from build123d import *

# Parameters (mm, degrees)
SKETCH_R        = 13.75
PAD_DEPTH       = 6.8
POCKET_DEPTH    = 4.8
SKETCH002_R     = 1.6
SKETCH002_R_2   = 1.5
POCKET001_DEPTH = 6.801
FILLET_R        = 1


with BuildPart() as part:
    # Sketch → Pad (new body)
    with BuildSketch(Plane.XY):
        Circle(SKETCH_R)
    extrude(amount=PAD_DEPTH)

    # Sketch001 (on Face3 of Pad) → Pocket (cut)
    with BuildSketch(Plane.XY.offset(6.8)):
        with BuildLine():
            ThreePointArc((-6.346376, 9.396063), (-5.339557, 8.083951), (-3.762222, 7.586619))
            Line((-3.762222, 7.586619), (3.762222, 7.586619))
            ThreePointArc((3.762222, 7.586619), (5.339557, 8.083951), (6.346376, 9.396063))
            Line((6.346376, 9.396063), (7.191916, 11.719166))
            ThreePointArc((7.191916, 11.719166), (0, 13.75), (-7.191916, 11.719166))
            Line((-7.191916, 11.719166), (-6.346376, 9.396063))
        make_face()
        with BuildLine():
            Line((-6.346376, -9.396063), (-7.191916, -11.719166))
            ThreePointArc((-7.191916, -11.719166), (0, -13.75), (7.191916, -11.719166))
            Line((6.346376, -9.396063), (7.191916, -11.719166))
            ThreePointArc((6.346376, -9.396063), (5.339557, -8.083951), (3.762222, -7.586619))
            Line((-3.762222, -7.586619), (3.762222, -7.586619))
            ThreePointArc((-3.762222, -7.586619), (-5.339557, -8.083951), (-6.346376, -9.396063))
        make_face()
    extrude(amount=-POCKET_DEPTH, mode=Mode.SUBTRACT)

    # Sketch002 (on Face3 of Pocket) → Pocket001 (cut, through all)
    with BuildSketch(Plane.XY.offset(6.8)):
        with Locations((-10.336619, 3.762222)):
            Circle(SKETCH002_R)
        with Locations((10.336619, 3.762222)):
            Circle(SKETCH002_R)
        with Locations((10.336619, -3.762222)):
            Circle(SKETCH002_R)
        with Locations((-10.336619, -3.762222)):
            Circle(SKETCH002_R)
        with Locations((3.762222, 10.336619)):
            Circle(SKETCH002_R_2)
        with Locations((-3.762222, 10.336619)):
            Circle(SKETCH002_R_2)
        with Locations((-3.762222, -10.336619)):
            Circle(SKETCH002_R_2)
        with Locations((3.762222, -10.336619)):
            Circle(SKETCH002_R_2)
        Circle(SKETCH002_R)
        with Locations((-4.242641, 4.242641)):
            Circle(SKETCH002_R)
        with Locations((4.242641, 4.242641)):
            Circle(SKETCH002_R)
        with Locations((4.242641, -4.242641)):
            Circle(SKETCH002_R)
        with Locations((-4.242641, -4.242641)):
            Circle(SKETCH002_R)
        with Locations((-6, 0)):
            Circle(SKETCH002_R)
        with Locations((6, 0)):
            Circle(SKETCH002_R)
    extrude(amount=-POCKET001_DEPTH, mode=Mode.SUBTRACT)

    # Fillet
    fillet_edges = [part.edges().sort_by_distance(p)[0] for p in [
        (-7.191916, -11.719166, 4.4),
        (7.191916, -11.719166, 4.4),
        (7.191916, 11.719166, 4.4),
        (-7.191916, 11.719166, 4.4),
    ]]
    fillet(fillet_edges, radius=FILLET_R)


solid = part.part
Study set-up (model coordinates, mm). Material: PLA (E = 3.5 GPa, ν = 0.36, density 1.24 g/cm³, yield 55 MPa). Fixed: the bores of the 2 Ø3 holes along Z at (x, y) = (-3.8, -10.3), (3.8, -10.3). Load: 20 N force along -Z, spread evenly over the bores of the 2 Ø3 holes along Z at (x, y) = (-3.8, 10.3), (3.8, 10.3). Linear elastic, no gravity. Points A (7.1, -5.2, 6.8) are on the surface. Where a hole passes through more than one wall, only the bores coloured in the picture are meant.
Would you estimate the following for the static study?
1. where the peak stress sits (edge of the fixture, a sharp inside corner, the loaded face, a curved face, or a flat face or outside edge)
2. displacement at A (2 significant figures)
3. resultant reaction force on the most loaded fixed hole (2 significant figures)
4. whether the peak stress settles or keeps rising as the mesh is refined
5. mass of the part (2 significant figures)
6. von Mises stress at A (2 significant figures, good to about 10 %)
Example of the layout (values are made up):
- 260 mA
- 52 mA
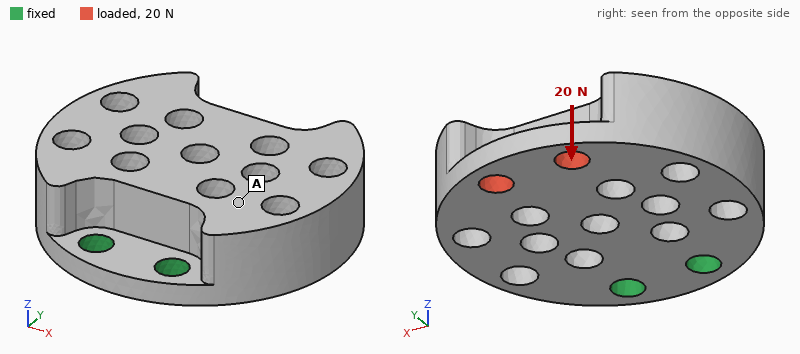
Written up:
- edge of the fixture
- 0.11 mm
- 11 N
- keeps rising
- 3.3 g
- 3.5 MPa
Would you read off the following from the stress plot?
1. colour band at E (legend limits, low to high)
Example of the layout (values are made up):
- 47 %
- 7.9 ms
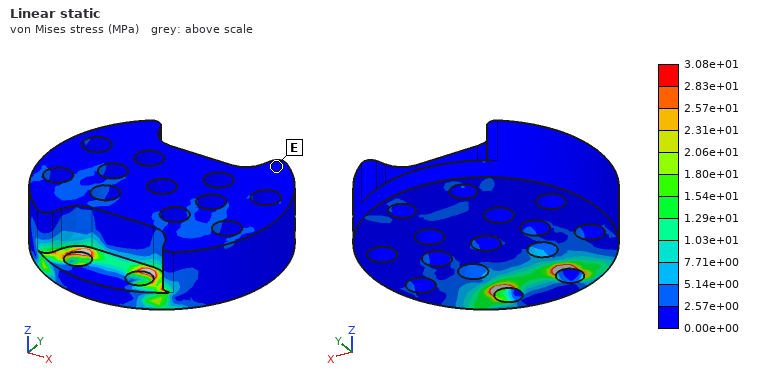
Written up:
- 0.00e+00 to 2.57e+00 MPa
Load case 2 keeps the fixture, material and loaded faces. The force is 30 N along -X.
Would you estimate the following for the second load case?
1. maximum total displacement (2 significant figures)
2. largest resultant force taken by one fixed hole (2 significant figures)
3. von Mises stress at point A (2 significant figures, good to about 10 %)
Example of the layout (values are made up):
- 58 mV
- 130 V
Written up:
- 64 µm
- 59 N
- 0.75 MPa
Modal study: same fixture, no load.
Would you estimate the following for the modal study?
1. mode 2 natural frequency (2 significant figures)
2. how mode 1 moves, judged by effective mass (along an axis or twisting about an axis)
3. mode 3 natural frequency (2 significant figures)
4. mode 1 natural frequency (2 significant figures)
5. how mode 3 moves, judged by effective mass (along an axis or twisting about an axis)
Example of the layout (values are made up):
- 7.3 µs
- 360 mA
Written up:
- 3000 Hz
- along Z
- 3700 Hz
- 1200 Hz
- along X
